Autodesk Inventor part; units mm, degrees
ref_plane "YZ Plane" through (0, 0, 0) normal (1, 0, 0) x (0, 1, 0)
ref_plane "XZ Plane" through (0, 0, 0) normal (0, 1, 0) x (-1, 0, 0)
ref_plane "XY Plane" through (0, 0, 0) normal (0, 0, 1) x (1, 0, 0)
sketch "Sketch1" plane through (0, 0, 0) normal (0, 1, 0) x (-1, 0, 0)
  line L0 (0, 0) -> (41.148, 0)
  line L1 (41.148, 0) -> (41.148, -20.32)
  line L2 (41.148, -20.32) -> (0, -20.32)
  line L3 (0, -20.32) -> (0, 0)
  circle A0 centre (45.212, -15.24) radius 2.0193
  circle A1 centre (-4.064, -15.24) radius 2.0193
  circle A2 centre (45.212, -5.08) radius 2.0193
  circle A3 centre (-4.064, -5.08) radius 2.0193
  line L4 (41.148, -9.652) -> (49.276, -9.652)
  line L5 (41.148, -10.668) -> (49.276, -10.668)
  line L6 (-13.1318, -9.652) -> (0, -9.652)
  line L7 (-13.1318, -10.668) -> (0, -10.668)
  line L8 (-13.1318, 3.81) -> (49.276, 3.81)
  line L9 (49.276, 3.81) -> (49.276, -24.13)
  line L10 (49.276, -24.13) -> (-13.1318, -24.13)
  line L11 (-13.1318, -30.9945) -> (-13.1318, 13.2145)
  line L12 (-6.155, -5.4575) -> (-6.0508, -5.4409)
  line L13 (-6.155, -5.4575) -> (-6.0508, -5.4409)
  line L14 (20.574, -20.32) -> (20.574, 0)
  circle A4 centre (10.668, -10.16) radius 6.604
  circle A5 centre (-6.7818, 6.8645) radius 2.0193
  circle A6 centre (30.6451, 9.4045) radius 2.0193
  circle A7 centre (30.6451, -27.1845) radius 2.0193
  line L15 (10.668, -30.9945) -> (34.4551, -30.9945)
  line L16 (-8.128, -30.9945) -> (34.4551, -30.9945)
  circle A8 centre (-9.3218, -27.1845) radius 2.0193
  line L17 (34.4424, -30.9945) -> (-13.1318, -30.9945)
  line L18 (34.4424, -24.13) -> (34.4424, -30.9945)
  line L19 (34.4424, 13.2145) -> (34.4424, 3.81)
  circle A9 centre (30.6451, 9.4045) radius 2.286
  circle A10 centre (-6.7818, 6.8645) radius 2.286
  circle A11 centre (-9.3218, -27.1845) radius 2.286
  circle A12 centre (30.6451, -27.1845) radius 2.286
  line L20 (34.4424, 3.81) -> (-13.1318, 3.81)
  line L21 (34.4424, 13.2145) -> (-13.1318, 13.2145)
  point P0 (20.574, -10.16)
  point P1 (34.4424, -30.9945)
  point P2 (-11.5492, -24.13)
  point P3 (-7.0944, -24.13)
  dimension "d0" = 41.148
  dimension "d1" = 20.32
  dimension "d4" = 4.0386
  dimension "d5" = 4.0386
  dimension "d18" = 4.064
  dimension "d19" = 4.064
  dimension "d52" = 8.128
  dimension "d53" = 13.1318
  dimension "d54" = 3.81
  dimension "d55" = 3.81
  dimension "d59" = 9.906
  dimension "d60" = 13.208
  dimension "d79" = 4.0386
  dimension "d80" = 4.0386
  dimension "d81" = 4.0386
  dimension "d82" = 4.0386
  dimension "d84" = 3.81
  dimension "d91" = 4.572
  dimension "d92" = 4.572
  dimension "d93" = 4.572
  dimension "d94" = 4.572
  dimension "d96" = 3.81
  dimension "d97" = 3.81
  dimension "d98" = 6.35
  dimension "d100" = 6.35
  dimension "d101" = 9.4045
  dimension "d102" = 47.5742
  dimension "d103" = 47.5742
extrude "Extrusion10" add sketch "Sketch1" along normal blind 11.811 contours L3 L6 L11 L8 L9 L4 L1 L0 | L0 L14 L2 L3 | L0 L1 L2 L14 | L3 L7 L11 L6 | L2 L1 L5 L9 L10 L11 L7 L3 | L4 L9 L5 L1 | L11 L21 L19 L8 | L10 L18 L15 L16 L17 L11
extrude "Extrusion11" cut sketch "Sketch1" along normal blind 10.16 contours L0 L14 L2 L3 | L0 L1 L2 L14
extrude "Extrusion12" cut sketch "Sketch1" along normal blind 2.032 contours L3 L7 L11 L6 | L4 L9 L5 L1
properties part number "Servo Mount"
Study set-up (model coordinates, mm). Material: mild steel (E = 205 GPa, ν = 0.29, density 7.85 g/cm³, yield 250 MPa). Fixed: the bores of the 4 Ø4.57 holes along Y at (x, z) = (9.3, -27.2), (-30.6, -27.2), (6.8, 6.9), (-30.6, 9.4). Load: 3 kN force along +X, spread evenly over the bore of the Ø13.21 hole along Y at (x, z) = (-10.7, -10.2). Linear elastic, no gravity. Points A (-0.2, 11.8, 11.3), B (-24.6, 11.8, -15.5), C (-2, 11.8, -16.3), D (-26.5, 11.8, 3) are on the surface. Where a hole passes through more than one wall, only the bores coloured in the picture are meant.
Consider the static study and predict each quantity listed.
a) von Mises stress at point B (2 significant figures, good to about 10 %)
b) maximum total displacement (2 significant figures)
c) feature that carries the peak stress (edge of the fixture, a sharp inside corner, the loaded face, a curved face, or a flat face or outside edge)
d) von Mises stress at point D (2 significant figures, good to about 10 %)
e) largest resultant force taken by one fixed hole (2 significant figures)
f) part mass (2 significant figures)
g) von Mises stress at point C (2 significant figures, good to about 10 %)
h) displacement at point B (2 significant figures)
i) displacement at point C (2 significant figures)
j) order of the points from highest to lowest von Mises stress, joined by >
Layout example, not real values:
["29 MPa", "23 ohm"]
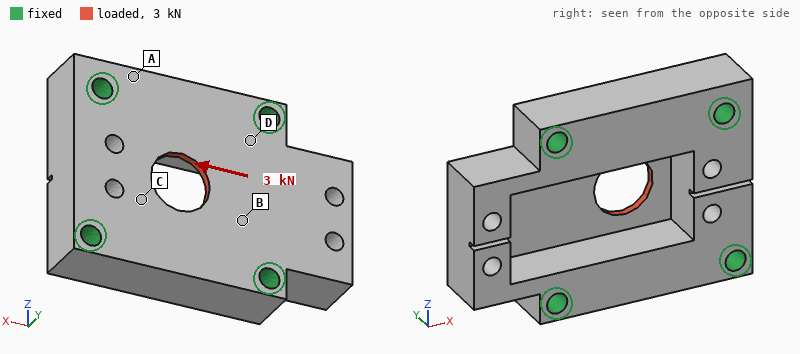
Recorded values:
["26 MPa", "3.4 µm", "the loaded face", "13 MPa", "910 N", "150 g", "38 MPa", "1.4 µm", "1.9 µm", "C > B > D > A"]
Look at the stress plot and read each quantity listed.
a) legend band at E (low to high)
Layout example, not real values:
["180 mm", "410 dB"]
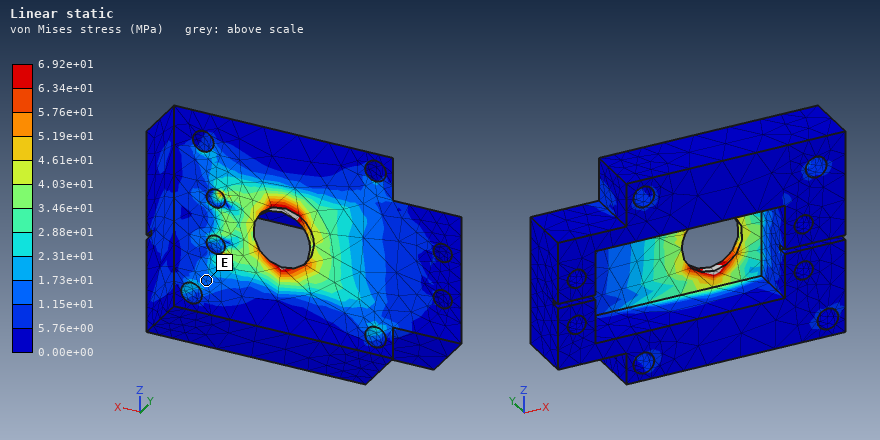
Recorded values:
["1.15e+01 to 1.73e+01 MPa"]
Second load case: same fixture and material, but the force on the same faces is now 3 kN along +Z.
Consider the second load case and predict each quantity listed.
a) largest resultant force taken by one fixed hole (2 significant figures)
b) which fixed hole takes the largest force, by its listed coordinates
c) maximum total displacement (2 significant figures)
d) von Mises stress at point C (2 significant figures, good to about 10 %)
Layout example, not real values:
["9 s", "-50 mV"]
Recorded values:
["1.0 kN", "(6.8, 6.9)", "4.2 µm", "35 MPa"]
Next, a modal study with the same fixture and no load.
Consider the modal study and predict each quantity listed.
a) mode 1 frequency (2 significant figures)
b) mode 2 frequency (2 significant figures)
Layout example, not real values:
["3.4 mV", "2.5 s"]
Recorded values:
["12 kHz", "17 kHz"]
